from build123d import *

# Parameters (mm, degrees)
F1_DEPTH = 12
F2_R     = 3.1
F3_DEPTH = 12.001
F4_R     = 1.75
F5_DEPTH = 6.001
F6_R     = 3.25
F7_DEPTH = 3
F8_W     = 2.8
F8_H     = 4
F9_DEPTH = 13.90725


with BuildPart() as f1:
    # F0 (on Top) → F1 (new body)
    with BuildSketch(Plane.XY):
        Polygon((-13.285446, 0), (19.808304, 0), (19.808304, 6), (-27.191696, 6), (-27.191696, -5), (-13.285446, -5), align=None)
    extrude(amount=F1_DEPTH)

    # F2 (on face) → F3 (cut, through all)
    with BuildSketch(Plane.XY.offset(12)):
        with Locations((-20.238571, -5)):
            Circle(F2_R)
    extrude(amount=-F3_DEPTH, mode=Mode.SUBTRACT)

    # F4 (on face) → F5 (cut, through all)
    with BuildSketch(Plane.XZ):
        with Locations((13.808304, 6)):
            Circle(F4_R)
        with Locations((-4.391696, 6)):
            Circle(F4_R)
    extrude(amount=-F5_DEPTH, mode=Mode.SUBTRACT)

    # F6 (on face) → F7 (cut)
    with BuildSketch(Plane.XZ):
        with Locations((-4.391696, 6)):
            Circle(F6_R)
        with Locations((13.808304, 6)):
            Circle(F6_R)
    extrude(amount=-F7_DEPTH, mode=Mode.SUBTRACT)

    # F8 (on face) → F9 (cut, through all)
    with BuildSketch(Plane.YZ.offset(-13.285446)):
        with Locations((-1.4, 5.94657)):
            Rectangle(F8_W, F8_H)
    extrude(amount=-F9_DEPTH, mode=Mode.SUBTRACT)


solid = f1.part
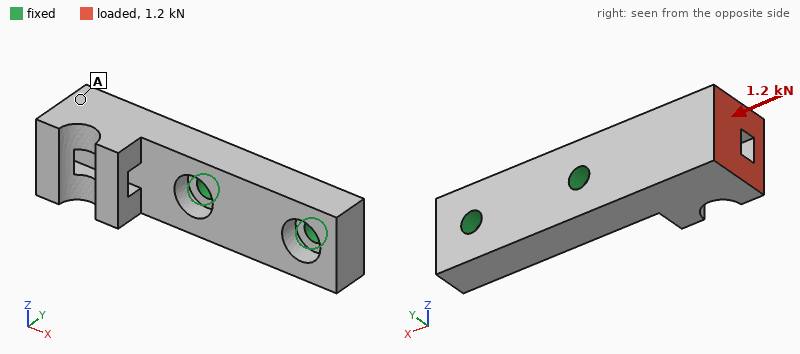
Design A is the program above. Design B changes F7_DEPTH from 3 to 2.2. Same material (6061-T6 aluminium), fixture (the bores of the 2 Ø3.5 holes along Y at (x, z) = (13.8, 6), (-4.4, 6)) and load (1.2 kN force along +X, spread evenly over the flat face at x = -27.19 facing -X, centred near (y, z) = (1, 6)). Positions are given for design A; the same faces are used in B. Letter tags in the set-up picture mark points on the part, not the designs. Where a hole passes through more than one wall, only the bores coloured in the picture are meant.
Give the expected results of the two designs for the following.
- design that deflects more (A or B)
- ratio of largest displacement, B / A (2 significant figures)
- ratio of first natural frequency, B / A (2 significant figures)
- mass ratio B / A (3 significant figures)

A
0.86
1.1
1.01
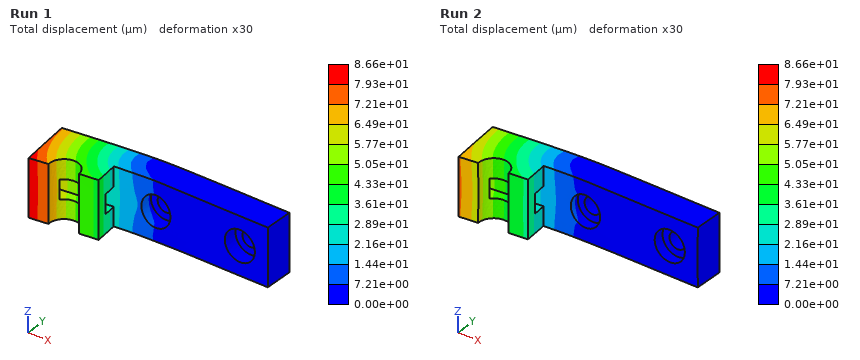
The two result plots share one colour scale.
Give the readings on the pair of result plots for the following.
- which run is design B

Run 2
